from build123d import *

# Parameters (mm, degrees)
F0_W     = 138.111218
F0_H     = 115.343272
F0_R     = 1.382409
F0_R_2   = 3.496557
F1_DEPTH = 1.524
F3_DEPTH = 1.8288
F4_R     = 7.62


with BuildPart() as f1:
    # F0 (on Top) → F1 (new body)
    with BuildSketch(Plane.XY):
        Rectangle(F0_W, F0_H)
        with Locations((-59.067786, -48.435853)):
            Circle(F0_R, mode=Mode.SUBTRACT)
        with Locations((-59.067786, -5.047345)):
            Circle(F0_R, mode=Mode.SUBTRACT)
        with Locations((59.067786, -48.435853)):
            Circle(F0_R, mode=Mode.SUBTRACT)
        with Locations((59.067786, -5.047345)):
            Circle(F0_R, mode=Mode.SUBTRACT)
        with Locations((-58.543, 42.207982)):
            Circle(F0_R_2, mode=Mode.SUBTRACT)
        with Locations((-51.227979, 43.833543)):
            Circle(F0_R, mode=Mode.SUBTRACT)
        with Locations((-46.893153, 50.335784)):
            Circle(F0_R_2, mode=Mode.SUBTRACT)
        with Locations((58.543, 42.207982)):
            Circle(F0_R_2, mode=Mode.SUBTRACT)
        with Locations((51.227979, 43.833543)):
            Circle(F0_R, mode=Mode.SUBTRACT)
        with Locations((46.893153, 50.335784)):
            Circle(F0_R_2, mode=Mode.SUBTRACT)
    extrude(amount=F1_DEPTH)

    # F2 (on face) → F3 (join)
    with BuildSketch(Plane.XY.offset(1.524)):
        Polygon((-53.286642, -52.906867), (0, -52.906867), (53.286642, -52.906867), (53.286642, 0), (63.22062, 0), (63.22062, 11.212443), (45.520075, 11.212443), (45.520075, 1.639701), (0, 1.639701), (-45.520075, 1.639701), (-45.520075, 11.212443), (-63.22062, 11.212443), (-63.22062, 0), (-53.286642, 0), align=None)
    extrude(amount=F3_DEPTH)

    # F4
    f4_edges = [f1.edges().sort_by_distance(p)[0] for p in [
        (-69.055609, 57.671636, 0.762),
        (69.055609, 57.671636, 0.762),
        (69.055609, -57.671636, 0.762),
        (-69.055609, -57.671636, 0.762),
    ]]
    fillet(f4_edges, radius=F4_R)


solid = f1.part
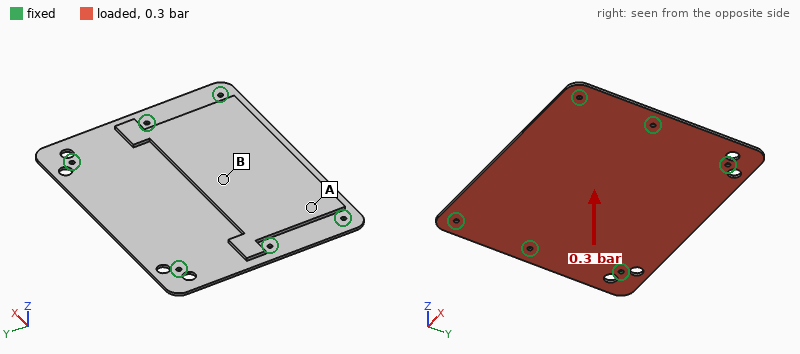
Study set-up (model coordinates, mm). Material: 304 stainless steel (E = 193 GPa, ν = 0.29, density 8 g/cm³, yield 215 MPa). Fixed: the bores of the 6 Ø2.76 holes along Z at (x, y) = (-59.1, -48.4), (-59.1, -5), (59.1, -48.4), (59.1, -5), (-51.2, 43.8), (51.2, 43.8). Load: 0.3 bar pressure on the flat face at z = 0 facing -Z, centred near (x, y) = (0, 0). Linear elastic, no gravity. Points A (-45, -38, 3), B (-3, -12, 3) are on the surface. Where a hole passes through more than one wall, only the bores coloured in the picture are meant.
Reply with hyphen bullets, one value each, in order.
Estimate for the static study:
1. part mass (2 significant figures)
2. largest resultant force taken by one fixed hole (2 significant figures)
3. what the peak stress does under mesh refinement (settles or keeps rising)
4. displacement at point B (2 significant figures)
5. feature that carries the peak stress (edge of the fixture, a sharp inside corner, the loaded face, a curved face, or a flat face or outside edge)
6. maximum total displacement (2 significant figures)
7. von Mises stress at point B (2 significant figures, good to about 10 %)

- 280 g
- 330 N
- keeps rising
- 0.082 mm
- edge of the fixture
- 0.18 mm
- 26 MPa
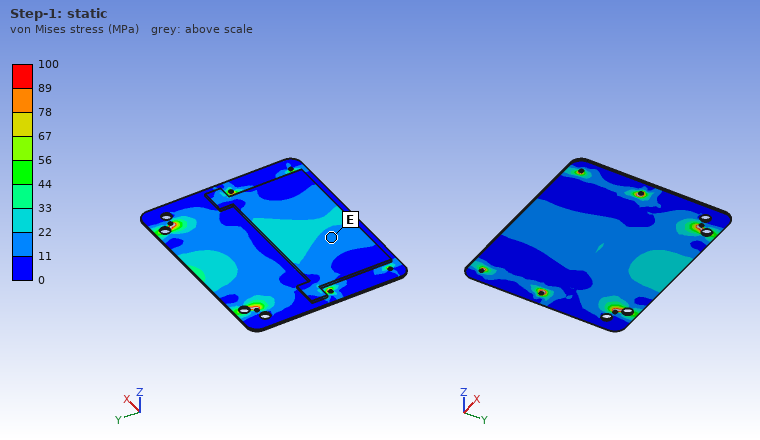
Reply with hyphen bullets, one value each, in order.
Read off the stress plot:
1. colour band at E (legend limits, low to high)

- 11 to 22 MPa
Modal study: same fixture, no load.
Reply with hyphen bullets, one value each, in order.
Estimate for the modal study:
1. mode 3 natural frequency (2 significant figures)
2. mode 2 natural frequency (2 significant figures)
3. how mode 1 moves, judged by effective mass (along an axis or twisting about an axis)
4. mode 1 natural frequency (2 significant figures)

- 1500 Hz
- 920 Hz
- along Z
- 720 Hz
